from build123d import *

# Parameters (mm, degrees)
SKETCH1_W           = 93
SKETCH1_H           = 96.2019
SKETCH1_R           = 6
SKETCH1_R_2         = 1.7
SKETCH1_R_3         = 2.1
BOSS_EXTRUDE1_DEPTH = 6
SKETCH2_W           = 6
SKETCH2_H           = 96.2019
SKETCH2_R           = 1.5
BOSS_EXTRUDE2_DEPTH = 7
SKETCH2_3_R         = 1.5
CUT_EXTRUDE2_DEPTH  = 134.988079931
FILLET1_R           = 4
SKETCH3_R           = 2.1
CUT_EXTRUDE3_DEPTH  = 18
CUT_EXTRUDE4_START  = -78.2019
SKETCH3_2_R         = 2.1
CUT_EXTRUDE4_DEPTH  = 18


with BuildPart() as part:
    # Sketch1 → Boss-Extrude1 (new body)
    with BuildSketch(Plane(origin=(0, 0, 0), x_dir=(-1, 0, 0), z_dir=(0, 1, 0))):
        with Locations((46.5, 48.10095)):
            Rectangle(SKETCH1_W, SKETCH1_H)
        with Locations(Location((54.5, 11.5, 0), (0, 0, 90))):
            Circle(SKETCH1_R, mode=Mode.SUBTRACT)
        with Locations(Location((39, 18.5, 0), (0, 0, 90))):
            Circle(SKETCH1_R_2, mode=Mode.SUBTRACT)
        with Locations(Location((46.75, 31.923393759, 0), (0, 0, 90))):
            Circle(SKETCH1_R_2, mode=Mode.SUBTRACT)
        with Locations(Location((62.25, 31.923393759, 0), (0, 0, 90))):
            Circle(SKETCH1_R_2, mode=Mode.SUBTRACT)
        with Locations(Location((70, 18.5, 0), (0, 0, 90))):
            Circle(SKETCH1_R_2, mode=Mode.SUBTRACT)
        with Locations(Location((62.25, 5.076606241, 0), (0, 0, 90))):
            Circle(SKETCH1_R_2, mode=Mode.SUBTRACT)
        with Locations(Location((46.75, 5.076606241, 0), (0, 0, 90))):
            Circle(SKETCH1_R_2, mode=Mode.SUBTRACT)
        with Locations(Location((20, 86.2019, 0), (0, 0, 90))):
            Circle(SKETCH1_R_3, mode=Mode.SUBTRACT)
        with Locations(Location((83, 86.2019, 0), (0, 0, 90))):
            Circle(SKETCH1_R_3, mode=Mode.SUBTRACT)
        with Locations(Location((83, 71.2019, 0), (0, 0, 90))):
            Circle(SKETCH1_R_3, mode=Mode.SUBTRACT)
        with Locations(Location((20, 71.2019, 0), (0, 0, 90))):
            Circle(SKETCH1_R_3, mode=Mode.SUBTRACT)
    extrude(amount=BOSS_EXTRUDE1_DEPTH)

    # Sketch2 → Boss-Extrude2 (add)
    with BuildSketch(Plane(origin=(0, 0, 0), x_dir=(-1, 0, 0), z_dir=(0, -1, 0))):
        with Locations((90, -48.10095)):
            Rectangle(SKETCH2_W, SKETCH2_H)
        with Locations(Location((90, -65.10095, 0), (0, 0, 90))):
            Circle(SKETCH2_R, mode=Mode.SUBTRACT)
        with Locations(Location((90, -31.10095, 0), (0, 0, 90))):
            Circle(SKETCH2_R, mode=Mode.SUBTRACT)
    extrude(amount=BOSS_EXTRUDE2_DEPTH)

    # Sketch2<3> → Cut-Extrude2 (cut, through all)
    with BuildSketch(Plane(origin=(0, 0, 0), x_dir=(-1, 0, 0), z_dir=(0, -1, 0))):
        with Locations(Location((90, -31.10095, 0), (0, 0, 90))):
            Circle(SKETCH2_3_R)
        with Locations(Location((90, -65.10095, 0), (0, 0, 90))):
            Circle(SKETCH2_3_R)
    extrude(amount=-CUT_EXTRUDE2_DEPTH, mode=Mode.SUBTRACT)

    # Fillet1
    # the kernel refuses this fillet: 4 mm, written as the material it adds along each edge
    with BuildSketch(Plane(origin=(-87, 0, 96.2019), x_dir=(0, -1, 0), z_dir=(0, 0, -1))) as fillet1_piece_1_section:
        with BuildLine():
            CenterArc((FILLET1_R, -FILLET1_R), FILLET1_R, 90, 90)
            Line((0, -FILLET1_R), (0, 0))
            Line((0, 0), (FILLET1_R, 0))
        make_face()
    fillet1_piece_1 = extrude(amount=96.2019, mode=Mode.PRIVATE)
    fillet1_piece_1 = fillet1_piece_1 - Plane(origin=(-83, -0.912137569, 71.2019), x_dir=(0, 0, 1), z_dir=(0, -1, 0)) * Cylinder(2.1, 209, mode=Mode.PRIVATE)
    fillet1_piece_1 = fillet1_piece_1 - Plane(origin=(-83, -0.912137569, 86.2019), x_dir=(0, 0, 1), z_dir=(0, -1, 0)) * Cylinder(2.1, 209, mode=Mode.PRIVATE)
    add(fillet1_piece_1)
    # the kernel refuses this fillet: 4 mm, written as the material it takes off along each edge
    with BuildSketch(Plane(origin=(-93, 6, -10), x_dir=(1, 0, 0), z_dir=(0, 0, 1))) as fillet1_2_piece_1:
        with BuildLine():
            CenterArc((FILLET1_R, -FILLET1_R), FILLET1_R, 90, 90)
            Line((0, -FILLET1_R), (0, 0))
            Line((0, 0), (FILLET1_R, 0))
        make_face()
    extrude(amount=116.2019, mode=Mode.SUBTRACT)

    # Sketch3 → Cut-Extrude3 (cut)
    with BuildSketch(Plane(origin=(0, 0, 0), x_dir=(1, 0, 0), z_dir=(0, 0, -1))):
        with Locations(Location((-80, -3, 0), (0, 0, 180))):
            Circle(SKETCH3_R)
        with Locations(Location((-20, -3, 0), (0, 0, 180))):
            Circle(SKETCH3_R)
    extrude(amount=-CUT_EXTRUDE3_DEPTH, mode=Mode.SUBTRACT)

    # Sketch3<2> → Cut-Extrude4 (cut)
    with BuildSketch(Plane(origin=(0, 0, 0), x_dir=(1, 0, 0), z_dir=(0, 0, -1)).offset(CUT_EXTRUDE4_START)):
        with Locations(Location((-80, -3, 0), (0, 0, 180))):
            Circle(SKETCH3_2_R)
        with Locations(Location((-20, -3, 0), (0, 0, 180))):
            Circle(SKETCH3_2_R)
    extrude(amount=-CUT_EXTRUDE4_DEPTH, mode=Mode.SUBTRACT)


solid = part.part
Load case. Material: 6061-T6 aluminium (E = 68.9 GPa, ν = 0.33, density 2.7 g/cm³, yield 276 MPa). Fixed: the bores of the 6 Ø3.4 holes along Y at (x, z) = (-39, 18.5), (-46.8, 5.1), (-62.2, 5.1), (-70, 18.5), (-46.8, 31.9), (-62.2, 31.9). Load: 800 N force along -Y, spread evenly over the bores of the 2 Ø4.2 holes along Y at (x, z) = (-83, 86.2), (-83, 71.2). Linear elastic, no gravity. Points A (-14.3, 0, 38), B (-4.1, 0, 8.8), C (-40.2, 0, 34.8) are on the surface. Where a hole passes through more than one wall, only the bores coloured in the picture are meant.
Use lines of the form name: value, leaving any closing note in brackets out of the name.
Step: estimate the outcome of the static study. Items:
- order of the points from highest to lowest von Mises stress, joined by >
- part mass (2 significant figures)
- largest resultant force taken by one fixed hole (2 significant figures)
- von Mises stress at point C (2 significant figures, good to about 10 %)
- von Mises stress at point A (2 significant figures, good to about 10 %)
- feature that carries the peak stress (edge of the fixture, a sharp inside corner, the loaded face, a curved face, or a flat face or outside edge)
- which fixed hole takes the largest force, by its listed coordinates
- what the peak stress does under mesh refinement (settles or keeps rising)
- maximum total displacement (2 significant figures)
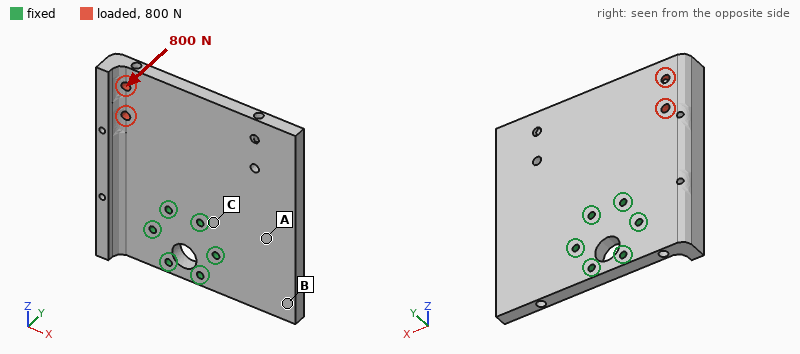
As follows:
order of the points from highest to lowest von Mises stress, joined by >: C > A > B
part mass: 150 g
largest resultant force taken by one fixed hole: 1.6 kN
von Mises stress at point C: 32 MPa
von Mises stress at point A: 17 MPa
feature that carries the peak stress: edge of the fixture
which fixed hole takes the largest force, by its listed coordinates: (-62.2, 31.9)
what the peak stress does under mesh refinement: keeps rising
maximum total displacement: 0.56 mm
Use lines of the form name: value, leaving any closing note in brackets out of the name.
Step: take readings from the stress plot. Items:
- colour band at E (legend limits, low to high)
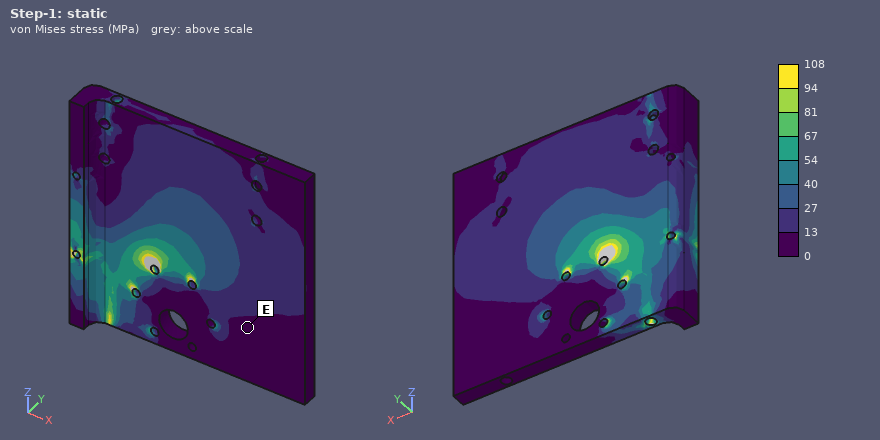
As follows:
colour band at E: 0 to 13 MPa
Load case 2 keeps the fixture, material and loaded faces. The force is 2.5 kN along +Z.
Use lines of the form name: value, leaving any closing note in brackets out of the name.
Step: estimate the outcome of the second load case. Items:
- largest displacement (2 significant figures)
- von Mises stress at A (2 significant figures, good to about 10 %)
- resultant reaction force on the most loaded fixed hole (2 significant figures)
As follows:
largest displacement: 39 µm
von Mises stress at A: 3.5 MPa
resultant reaction force on the most loaded fixed hole: 1.5 kN
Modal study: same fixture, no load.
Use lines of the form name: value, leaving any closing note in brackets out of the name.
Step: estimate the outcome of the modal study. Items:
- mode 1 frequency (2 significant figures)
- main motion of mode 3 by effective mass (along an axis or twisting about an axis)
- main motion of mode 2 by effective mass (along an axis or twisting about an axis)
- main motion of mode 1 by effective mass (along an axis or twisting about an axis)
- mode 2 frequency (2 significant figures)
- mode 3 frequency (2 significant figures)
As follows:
mode 1 frequency: 1100 Hz
main motion of mode 3 by effective mass: along Y
main motion of mode 2 by effective mass: twisting about Z
main motion of mode 1 by effective mass: along Y
mode 2 frequency: 1500 Hz
mode 3 frequency: 3000 Hz
